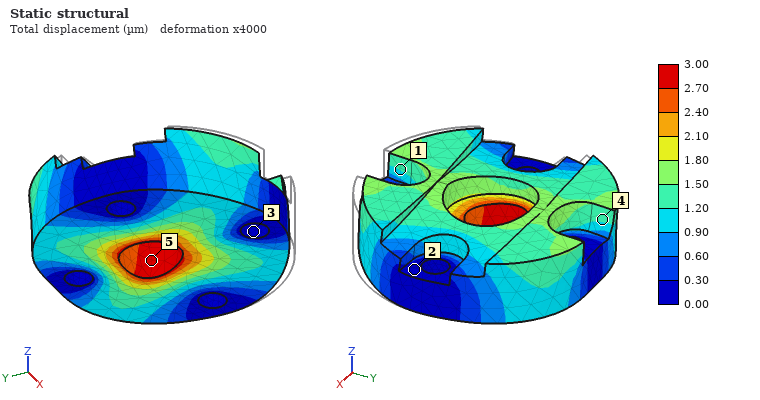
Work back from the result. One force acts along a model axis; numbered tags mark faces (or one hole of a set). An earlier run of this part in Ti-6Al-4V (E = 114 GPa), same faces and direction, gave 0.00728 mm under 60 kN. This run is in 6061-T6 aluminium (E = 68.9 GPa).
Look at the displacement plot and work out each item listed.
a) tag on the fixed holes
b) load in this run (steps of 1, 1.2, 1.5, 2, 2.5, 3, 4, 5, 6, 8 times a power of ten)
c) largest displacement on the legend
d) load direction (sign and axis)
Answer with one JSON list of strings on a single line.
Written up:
["3", "15 kN", "3.00 µm", "+Y"]
